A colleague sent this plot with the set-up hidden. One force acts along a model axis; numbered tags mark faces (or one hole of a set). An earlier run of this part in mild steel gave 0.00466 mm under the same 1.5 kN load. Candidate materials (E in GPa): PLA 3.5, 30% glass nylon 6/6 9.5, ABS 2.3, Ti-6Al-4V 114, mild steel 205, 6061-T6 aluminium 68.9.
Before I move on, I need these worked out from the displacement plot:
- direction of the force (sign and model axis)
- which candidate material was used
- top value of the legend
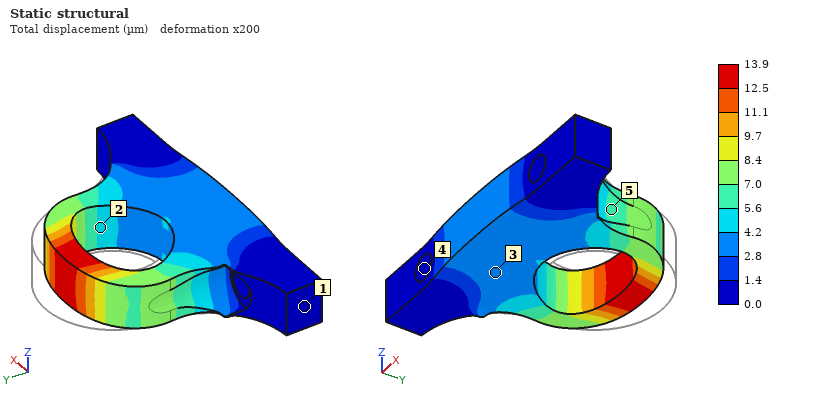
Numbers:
-Y
6061-T6 aluminium
13.9 µm
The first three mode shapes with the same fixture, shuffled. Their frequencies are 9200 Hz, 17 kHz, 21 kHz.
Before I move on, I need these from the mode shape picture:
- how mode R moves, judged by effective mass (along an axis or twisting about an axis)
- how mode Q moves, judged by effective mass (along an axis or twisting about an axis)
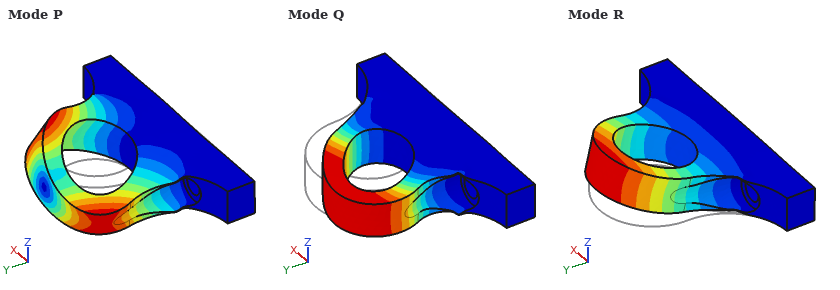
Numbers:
along Z
along X
